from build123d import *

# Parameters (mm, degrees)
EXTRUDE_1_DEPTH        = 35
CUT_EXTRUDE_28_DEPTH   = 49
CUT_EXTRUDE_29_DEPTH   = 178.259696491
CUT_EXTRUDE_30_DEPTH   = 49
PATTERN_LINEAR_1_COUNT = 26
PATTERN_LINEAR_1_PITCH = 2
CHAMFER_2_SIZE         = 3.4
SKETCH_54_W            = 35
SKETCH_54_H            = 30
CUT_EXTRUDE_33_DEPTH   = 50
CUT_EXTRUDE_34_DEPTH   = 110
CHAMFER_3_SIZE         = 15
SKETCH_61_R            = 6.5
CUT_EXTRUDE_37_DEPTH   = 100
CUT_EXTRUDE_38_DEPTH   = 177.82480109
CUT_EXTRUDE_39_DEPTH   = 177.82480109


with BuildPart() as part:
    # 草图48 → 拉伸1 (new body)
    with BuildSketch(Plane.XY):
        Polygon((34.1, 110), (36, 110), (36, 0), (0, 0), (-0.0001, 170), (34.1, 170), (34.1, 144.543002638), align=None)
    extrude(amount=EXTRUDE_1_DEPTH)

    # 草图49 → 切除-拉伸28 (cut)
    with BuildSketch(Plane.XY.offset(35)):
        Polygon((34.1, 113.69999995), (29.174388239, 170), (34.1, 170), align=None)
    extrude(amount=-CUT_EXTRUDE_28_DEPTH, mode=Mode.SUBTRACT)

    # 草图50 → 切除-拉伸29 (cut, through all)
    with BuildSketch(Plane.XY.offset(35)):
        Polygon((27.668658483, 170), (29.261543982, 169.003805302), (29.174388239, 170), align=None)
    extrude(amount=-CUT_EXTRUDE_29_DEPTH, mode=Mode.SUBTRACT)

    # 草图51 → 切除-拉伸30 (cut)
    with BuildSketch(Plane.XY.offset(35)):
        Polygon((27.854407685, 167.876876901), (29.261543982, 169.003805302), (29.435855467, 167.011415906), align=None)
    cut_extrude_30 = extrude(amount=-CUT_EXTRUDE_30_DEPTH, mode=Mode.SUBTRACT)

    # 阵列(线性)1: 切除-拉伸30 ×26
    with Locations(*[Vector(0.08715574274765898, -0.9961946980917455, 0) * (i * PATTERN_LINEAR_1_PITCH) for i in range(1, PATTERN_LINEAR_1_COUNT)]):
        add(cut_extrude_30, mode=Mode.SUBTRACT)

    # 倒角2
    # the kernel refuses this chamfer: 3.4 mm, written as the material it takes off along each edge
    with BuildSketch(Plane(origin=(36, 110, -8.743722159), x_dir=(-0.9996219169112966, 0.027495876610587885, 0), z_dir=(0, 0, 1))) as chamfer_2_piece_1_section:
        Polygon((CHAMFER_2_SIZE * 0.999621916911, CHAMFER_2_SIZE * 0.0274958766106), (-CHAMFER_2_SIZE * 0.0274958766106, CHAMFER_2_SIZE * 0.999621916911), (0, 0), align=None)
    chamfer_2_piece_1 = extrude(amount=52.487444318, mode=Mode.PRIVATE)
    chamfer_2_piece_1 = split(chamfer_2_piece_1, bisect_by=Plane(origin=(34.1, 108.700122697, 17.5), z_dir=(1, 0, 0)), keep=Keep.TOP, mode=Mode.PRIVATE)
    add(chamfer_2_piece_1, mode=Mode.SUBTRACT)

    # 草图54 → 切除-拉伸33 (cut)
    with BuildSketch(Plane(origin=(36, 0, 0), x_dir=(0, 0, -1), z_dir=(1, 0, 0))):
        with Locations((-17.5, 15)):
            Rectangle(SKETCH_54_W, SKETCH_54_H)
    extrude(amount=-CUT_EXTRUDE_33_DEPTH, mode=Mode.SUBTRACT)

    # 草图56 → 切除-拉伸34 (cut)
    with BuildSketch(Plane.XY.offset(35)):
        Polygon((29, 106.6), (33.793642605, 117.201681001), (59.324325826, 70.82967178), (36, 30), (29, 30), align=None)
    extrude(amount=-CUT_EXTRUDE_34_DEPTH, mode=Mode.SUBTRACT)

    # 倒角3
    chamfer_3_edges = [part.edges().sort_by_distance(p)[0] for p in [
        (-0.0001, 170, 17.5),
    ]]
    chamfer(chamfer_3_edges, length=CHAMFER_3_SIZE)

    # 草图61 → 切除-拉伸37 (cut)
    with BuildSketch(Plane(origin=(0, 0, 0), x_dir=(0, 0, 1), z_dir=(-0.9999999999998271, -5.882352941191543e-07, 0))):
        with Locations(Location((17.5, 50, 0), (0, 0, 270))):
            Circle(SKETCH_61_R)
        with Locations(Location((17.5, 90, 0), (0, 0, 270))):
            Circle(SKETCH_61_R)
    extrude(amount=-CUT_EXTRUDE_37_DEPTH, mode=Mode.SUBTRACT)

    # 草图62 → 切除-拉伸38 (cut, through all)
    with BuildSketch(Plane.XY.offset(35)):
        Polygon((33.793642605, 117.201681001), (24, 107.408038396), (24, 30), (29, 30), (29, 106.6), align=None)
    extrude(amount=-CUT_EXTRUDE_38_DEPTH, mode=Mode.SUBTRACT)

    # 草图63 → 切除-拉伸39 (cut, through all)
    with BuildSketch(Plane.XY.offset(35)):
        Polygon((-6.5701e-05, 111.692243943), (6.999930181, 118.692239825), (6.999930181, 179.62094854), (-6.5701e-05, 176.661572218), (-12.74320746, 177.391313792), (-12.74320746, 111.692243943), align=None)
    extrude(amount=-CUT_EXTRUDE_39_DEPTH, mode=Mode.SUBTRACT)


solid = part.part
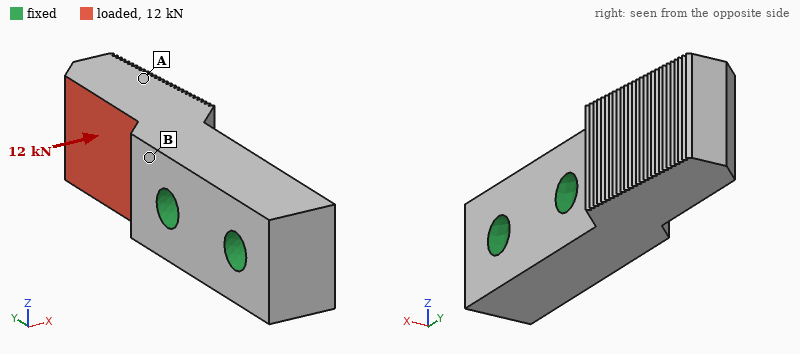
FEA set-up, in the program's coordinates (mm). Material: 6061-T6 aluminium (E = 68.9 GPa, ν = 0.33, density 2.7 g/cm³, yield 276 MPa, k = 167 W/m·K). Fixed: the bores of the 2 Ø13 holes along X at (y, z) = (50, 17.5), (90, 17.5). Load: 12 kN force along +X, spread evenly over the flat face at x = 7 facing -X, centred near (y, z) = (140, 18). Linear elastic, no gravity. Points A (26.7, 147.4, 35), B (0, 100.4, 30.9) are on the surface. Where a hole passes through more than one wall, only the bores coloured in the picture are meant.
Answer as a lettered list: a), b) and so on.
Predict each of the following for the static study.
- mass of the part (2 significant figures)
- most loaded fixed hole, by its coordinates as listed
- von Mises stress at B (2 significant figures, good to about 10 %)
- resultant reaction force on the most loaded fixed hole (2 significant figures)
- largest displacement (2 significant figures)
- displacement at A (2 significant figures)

a) 300 g
b) (90, 17.5)
c) 100 MPa
d) 14 kN
e) 0.39 mm
f) 0.26 mm
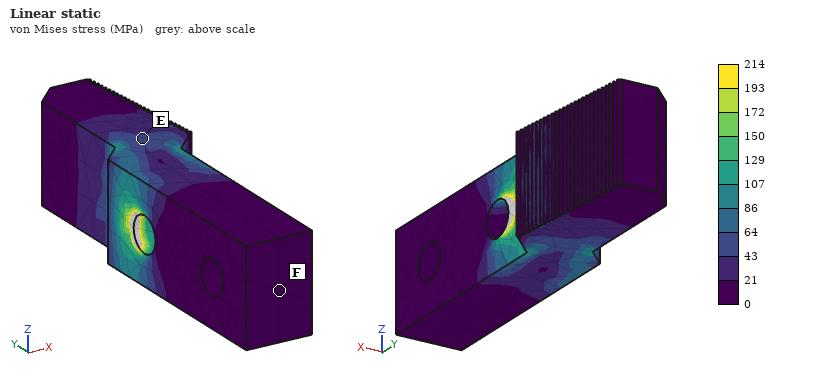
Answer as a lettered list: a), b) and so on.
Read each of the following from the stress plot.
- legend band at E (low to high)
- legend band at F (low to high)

a) 43 to 64 MPa
b) 0 to 21 MPa
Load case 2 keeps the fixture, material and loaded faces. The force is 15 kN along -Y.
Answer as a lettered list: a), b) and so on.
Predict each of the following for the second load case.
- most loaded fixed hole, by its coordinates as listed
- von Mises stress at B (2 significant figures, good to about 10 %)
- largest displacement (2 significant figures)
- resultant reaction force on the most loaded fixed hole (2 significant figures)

a) (90, 17.5)
b) 27 MPa
c) 0.12 mm
d) 14 kN
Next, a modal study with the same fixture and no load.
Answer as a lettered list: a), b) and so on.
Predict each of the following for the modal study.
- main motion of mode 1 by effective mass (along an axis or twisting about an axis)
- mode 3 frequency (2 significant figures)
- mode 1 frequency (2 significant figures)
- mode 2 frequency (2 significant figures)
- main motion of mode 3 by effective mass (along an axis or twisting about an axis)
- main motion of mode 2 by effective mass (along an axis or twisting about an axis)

a) along X
b) 8800 Hz
c) 3000 Hz
d) 3600 Hz
e) twisting about Y
f) along Z
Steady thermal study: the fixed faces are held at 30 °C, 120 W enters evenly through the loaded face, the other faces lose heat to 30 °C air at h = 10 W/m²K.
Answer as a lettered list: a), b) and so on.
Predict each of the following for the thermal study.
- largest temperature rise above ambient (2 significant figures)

a) 44 K
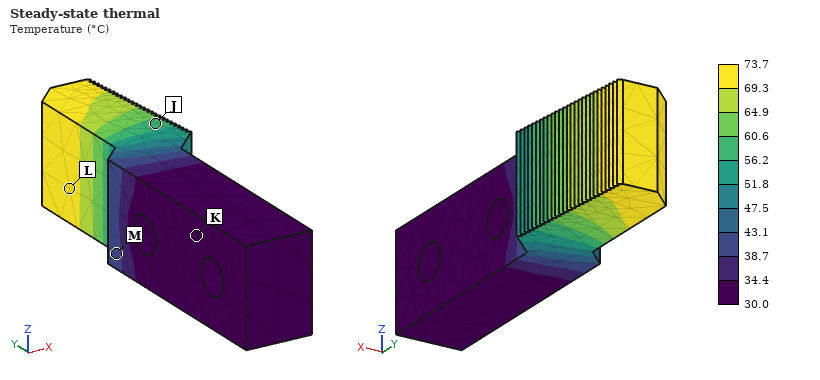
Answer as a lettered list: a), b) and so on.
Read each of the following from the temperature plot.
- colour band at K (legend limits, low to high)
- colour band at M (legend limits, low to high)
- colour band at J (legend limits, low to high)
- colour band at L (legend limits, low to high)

a) 30.0 to 34.4 °C
b) 38.7 to 43.1 °C
c) 56.2 to 60.6 °C
d) 69.3 to 73.7 °C
